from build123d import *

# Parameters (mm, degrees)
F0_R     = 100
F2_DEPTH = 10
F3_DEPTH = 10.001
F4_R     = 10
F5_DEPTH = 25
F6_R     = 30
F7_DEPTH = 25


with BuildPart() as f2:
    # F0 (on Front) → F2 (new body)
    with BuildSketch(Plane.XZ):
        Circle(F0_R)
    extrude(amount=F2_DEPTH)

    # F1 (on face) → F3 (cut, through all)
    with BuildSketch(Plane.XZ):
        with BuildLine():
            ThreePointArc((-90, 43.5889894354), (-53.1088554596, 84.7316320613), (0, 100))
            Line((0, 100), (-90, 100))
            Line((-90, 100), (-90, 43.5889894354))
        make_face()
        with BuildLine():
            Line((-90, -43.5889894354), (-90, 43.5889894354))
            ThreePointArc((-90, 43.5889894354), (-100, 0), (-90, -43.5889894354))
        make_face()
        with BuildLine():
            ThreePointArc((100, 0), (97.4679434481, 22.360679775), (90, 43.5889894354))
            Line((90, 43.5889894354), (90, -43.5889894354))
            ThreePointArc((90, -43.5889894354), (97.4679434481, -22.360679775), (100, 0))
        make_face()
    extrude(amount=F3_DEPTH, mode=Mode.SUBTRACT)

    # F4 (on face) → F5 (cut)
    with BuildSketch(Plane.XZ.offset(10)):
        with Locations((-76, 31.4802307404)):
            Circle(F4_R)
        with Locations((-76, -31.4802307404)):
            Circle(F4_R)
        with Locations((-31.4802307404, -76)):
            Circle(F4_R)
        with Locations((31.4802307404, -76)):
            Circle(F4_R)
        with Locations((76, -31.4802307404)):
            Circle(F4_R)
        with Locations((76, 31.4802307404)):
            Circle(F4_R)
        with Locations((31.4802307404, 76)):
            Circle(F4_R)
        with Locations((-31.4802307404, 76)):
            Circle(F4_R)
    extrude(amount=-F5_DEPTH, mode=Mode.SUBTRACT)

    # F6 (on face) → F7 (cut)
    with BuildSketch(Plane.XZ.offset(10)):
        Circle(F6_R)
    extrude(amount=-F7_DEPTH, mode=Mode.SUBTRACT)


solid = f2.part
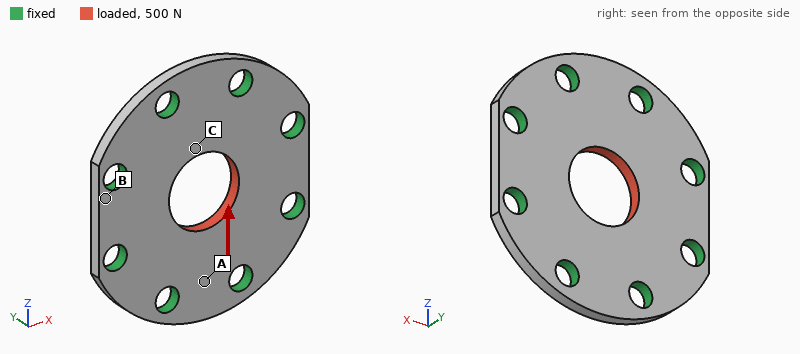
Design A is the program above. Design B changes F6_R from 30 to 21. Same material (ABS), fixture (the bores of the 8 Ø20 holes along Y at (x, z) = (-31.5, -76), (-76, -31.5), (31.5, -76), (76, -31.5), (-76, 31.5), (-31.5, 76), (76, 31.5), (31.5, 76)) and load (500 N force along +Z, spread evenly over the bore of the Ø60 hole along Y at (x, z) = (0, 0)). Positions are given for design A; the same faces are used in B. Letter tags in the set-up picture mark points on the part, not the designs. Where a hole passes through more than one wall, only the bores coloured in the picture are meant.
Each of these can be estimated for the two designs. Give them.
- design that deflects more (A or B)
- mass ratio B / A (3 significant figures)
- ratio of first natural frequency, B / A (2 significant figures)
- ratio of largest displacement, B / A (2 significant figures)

B
1.06
0.84
1.4
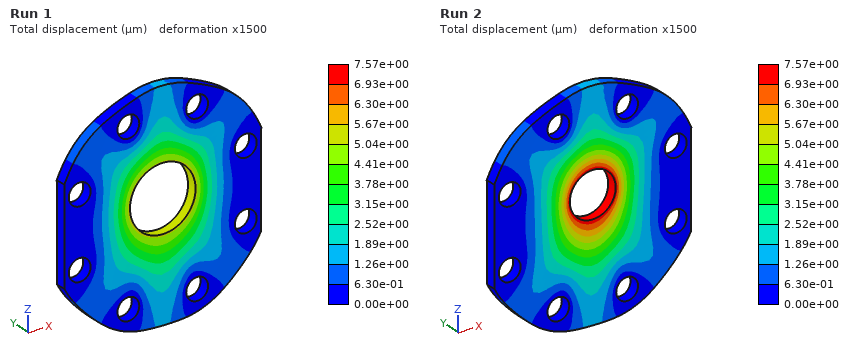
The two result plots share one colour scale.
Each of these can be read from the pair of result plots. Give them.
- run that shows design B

Run 2
